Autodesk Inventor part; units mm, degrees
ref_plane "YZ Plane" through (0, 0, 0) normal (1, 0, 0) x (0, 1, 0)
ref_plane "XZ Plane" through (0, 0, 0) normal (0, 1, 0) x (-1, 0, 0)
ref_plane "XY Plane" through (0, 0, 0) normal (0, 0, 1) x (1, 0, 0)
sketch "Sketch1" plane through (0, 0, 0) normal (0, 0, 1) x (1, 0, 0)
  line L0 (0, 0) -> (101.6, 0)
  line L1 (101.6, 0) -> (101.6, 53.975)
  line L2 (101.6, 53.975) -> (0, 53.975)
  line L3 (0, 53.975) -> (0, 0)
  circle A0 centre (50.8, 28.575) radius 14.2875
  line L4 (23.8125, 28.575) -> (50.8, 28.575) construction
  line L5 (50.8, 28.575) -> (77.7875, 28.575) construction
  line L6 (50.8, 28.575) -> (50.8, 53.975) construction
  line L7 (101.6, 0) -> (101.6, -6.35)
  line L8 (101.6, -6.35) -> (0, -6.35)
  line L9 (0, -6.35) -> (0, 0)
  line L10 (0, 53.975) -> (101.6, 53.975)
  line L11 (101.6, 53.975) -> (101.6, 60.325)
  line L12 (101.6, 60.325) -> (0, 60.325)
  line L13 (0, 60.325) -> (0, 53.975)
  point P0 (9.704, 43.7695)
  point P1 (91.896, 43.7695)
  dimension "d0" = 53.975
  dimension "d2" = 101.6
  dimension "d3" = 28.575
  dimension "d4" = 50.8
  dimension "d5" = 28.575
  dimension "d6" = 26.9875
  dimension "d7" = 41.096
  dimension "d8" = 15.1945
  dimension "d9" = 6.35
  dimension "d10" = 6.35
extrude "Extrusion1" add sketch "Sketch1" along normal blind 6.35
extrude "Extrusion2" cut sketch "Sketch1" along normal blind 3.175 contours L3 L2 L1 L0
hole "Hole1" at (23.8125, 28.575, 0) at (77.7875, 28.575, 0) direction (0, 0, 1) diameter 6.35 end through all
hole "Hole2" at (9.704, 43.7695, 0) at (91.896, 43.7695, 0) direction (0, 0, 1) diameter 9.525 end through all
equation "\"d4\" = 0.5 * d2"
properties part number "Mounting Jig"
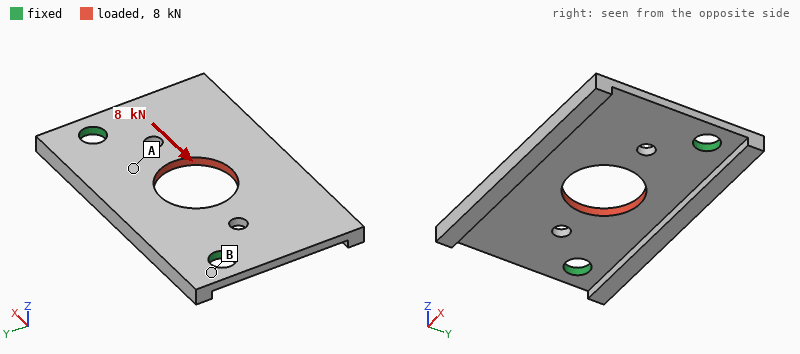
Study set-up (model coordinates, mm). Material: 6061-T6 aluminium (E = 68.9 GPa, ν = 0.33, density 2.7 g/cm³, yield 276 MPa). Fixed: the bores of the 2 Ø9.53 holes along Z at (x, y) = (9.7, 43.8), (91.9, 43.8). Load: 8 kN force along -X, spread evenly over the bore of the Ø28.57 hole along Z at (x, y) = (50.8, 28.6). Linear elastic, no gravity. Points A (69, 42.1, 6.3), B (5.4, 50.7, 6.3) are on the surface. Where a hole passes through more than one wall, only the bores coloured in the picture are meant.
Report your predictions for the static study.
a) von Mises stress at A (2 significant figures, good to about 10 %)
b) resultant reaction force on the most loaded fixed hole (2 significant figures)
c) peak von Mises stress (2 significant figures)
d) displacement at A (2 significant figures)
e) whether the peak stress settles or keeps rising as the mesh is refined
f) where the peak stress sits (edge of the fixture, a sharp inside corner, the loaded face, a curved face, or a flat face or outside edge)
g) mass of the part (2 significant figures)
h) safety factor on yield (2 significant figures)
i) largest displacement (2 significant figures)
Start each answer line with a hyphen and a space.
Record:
- 34 MPa
- 4.2 kN
- 140 MPa
- 12 µm
- settles
- a curved face
- 62 g
- 1.9
- 50 µm
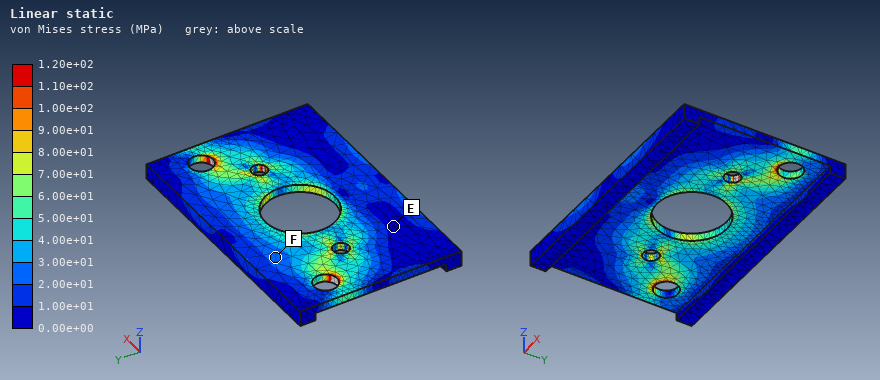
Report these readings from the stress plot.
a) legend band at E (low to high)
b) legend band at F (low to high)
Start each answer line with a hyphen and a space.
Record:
- 0.00e+00 to 1.00e+01 MPa
- 2.00e+01 to 3.00e+01 MPa
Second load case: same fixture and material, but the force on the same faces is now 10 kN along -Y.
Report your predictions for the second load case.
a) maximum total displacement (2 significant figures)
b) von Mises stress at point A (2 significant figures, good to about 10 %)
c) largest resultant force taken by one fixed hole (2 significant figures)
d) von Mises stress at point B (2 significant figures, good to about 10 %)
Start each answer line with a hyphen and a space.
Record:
- 98 µm
- 32 MPa
- 5.1 kN
- 31 MPa
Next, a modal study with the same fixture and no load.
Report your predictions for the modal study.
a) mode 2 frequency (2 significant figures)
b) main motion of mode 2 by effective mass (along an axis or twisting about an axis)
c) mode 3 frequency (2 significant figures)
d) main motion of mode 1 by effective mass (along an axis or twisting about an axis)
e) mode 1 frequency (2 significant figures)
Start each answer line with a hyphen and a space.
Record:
- 1600 Hz
- twisting about Y
- 3200 Hz
- along Z
- 770 Hz
